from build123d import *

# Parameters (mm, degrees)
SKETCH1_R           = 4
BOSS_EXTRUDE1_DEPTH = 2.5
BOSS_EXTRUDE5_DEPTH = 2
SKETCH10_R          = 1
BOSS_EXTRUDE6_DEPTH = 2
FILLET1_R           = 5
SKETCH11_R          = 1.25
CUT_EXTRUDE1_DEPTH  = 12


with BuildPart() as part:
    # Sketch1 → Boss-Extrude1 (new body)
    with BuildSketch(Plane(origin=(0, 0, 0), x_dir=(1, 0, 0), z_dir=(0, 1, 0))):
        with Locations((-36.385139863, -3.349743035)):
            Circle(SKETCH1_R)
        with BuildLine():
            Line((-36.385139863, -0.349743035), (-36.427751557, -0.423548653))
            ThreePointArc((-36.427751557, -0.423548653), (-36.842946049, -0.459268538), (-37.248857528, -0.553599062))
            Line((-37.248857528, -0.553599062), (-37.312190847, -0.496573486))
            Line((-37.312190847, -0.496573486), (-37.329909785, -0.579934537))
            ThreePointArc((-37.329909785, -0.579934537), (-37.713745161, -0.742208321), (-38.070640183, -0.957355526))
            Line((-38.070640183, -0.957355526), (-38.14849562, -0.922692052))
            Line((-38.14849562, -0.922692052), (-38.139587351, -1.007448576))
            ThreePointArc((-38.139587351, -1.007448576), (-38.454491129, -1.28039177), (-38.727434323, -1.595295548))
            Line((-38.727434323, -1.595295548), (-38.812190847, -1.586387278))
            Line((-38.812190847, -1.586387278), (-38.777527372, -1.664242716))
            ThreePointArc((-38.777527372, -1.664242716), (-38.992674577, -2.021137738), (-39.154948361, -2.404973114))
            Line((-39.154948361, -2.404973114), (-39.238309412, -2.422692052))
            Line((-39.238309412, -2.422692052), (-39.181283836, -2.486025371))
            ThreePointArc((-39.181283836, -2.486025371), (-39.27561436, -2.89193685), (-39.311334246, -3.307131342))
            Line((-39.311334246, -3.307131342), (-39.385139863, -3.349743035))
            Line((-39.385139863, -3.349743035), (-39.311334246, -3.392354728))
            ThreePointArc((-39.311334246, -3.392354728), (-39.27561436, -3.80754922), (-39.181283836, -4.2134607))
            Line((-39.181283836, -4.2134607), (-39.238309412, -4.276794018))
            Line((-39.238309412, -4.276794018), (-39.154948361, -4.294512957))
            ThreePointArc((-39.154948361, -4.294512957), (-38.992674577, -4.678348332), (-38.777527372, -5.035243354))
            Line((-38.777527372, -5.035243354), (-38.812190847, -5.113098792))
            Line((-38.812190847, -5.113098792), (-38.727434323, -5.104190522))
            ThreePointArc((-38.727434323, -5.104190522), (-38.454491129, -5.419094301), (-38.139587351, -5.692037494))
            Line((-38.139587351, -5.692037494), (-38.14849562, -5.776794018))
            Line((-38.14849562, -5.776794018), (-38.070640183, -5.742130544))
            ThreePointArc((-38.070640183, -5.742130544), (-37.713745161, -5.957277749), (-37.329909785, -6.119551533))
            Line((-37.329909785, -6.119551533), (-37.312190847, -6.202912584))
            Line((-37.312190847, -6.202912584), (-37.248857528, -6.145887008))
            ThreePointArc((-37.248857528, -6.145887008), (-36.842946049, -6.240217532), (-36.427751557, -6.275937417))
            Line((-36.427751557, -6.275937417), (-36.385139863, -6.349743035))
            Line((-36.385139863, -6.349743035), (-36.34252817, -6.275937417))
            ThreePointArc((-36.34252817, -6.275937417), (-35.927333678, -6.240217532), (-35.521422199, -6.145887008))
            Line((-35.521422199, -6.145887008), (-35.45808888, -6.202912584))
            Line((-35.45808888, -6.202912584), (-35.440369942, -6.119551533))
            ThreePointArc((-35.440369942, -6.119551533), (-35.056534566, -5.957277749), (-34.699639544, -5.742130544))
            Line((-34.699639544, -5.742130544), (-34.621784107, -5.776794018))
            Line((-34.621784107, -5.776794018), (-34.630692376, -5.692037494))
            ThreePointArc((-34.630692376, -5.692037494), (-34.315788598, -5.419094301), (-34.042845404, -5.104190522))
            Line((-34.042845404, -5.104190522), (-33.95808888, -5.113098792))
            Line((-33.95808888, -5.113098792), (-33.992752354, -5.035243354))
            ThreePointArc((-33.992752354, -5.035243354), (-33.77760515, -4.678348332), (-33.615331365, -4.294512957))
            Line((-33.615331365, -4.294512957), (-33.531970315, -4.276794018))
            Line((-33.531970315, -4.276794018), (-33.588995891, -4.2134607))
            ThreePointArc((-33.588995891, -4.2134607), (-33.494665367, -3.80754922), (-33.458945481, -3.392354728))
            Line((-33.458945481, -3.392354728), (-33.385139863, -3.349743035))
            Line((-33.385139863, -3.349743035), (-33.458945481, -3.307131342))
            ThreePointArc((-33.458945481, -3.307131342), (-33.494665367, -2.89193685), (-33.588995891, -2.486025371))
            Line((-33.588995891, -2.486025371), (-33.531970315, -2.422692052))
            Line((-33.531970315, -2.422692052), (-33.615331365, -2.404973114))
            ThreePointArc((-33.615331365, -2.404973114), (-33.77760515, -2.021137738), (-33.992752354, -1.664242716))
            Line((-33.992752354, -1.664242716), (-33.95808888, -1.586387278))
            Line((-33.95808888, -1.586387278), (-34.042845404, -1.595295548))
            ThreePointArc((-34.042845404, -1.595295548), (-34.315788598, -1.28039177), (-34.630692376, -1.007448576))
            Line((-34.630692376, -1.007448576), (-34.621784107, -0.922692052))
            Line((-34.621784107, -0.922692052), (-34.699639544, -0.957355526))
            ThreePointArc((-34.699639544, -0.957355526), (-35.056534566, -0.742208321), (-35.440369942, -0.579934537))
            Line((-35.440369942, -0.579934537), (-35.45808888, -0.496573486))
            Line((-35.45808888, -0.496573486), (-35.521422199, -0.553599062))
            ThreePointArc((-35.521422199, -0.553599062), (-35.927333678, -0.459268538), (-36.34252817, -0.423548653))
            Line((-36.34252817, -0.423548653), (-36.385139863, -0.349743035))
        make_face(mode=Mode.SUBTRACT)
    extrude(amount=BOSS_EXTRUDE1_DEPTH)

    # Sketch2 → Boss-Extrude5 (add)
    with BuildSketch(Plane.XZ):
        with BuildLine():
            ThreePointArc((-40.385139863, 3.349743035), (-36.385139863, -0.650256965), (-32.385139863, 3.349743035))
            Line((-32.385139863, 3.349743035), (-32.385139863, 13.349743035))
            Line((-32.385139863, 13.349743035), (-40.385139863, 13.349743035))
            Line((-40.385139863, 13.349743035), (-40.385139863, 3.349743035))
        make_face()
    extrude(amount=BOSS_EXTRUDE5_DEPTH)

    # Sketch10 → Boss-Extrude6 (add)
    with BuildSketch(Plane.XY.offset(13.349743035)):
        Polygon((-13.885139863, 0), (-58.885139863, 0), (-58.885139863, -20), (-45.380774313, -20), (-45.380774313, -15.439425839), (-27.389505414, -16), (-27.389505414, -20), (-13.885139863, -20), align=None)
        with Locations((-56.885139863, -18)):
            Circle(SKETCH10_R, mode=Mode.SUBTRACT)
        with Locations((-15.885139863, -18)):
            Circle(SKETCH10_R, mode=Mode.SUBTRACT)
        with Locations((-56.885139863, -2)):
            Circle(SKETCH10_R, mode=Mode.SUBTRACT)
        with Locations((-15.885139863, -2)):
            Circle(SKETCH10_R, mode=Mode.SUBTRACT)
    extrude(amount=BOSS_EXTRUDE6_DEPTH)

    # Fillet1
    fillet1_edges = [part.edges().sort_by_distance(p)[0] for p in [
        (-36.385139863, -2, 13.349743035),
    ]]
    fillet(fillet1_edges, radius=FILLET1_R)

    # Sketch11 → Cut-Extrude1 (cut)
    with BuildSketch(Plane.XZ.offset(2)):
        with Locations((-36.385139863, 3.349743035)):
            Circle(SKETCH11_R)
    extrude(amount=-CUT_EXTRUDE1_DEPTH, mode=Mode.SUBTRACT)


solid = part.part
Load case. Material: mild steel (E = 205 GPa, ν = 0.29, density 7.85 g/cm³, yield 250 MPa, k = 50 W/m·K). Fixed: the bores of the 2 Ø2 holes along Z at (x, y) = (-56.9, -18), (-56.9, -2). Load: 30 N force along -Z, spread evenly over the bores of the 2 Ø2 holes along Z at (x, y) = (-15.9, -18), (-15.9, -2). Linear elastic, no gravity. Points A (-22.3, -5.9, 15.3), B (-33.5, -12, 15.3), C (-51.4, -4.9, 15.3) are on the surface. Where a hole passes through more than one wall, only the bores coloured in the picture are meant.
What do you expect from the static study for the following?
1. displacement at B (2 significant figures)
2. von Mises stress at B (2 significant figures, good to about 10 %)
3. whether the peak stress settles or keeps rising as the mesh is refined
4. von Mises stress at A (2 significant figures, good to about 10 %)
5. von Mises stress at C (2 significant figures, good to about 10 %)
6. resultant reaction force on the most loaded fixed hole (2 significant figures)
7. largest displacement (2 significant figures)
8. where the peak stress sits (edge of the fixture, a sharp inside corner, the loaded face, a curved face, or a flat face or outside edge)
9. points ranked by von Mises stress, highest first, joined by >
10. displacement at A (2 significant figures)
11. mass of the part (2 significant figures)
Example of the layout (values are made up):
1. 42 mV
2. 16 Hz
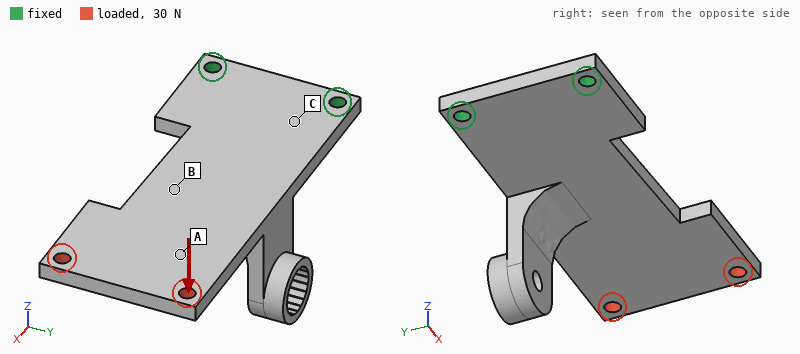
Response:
1. 0.12 mm
2. 42 MPa
3. keeps rising
4. 16 MPa
5. 82 MPa
6. 15 N
7. 0.31 mm
8. edge of the fixture
9. C > B > A
10. 0.22 mm
11. 15 g
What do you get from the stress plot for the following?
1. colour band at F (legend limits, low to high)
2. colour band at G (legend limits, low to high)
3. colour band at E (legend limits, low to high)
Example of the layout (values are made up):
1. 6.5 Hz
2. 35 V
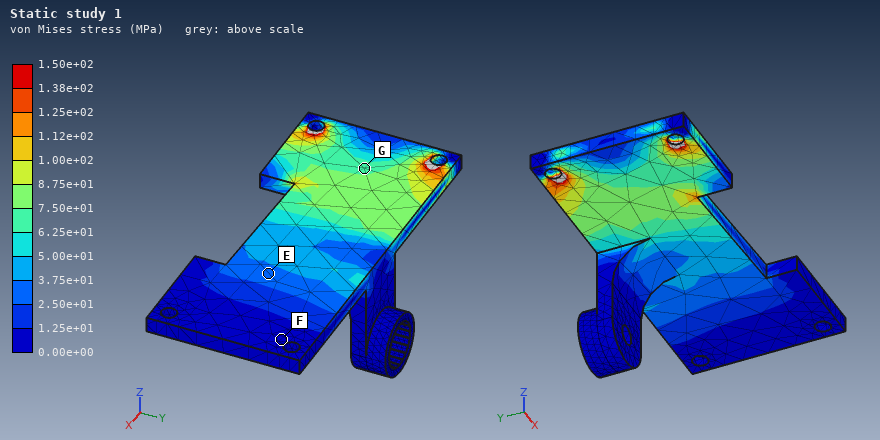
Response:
1. 0.00e+00 to 1.25e+01 MPa
2. 6.25e+01 to 7.50e+01 MPa
3. 2.50e+01 to 3.75e+01 MPa
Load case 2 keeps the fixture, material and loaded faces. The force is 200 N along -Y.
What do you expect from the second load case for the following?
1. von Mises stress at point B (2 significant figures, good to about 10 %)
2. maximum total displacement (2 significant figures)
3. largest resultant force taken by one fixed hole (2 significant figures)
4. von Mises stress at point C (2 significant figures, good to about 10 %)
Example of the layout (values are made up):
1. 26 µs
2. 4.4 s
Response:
1. 22 MPa
2. 35 µm
3. 520 N
4. 25 MPa
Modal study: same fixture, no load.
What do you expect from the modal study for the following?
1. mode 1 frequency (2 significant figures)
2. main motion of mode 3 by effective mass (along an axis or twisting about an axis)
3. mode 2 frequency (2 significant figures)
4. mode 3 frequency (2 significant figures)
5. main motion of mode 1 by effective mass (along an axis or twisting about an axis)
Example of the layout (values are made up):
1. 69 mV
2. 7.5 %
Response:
1. 810 Hz
2. along Z
3. 3100 Hz
4. 5300 Hz
5. along Z
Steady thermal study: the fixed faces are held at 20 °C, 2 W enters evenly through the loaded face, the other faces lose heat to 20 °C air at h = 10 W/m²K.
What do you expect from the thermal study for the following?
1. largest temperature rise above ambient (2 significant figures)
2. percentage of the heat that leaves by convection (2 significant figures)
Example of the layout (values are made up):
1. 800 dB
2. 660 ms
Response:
1. 46 K
2. 23 %
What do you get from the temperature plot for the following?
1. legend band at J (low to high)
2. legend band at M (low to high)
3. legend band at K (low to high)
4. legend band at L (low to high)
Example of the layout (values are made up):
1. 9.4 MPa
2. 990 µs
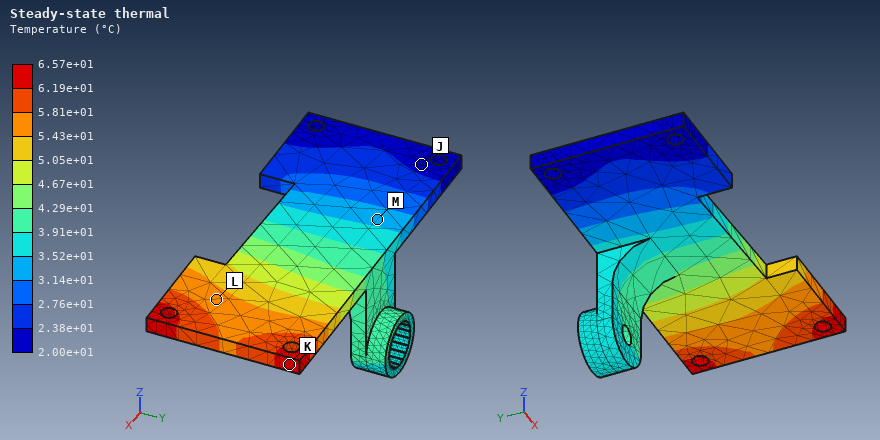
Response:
1. 2.00e+01 to 2.38e+01 °C
2. 3.14e+01 to 3.52e+01 °C
3. 6.19e+01 to 6.57e+01 °C
4. 5.43e+01 to 5.81e+01 °C
